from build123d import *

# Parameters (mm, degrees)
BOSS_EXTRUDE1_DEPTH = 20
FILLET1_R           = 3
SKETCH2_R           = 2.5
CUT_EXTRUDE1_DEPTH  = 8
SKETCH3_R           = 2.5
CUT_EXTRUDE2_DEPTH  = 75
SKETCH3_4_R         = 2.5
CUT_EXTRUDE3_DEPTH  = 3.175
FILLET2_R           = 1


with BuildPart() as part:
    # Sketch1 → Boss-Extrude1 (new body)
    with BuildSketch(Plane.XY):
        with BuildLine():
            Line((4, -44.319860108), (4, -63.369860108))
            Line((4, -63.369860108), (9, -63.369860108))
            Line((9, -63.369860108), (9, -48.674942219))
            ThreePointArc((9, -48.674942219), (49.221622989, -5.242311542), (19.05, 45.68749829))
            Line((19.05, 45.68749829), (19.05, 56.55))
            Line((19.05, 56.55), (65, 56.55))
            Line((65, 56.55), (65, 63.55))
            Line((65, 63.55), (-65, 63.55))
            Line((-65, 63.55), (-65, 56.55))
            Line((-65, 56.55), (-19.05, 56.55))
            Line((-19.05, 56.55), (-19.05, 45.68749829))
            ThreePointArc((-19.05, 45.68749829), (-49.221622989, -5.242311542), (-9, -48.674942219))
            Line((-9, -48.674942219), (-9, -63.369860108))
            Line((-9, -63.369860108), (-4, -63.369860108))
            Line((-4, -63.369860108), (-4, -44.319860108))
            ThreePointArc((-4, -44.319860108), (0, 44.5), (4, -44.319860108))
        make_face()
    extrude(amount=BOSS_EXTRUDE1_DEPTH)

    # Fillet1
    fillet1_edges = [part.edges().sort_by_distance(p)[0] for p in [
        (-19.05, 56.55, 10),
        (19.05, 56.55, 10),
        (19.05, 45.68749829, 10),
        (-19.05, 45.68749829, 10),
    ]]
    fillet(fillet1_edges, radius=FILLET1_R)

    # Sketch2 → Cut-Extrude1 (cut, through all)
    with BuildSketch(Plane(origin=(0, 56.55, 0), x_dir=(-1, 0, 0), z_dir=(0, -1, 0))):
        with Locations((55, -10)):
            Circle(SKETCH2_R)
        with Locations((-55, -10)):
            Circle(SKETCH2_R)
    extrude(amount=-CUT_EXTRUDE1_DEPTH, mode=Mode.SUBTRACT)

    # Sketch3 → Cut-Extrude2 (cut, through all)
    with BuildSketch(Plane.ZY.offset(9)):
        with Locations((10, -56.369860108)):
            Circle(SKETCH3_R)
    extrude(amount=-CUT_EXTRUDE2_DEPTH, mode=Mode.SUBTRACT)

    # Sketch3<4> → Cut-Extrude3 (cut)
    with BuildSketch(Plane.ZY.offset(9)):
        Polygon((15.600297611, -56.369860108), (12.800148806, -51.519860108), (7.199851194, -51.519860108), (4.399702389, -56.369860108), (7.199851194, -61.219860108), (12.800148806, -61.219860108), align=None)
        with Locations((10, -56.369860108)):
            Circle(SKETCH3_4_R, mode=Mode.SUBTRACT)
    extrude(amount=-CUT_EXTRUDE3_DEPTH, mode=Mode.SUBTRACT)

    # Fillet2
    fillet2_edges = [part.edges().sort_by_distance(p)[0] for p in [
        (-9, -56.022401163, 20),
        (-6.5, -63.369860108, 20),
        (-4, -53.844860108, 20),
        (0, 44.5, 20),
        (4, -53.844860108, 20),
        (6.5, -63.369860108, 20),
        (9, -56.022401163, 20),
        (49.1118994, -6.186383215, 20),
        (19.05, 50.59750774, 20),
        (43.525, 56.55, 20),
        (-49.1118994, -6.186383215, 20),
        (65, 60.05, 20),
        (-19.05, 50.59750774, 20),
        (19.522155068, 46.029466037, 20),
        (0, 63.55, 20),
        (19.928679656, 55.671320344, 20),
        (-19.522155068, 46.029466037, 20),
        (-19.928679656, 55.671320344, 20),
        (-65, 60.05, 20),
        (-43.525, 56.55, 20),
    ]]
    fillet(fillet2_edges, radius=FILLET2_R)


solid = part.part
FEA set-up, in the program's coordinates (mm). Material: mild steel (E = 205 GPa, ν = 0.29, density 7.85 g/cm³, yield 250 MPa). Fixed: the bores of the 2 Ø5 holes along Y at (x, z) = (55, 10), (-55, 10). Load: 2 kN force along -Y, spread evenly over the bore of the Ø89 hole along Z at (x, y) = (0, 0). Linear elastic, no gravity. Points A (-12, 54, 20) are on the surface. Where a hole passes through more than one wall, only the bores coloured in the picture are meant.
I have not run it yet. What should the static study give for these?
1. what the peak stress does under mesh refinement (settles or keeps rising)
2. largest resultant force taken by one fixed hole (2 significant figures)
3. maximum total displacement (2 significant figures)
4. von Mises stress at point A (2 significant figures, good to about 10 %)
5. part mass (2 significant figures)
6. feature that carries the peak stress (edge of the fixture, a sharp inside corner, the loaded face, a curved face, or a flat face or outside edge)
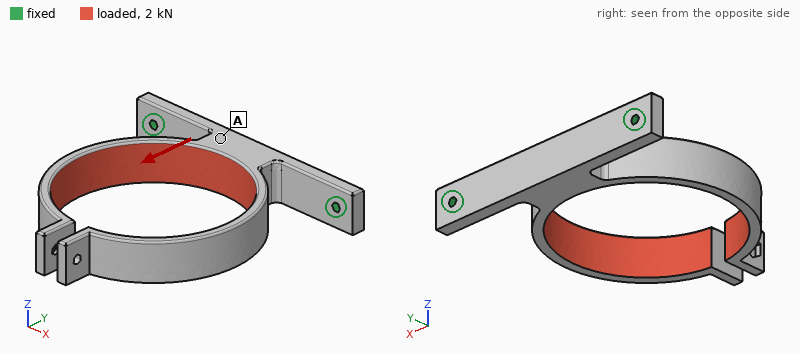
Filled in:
keeps rising
1.1 kN
0.54 mm
23 MPa
430 g
edge of the fixture
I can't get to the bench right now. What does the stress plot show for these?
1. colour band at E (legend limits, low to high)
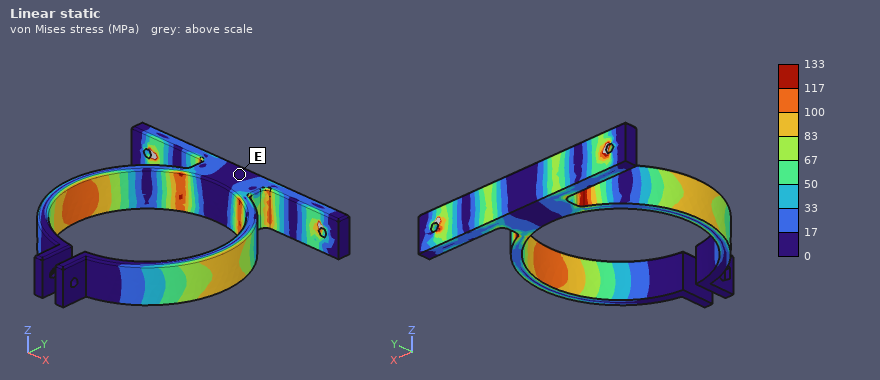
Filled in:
0 to 17 MPa
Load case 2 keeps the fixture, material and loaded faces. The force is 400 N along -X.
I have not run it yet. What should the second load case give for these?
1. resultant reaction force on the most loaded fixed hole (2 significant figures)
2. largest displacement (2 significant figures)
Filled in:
360 N
0.87 mm
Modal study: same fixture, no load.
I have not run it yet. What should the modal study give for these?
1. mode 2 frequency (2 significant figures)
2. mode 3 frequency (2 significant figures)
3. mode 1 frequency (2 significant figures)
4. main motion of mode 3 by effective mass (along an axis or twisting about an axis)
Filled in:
250 Hz
280 Hz
240 Hz
along Z
